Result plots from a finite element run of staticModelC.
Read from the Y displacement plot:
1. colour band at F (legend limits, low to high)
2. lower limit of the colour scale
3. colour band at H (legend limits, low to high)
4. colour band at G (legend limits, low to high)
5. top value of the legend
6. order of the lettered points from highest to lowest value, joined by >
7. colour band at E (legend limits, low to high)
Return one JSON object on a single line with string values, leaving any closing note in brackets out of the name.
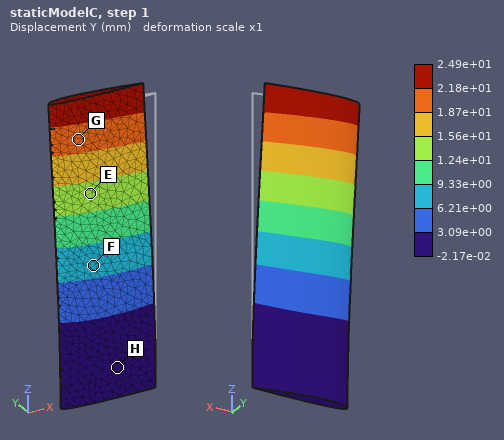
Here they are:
{"colour band at F": "6.21e+00 to 9.33e+00 mm", "lower limit of the colour scale": "-2.17e-02 mm", "colour band at H": "-2.17e-02 to 3.09e+00 mm", "colour band at G": "1.87e+01 to 2.18e+01 mm", "top value of the legend": "2.49e+01 mm", "order of the lettered points from highest to lowest value, joined by >": "G > E > F > H", "colour band at E": "1.24e+01 to 1.56e+01 mm"}
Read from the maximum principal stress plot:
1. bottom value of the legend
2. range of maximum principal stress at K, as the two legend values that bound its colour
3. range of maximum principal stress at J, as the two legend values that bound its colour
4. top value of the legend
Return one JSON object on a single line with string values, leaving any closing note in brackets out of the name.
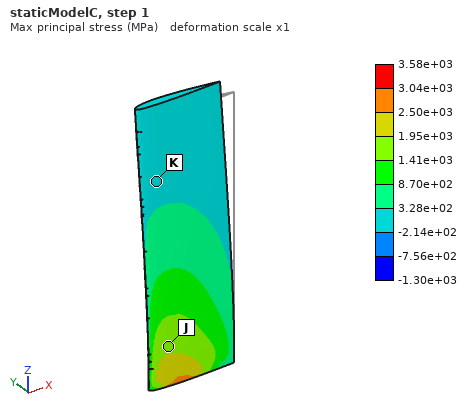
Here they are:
{"bottom value of the legend": "-1.30e+03 MPa", "range of maximum principal stress at K, as the two legend values that bound its colour": "-2.14e+02 to 3.28e+02 MPa", "range of maximum principal stress at J, as the two legend values that bound its colour": "1.41e+03 to 1.95e+03 MPa", "top value of the legend": "3.58e+03 MPa"}
